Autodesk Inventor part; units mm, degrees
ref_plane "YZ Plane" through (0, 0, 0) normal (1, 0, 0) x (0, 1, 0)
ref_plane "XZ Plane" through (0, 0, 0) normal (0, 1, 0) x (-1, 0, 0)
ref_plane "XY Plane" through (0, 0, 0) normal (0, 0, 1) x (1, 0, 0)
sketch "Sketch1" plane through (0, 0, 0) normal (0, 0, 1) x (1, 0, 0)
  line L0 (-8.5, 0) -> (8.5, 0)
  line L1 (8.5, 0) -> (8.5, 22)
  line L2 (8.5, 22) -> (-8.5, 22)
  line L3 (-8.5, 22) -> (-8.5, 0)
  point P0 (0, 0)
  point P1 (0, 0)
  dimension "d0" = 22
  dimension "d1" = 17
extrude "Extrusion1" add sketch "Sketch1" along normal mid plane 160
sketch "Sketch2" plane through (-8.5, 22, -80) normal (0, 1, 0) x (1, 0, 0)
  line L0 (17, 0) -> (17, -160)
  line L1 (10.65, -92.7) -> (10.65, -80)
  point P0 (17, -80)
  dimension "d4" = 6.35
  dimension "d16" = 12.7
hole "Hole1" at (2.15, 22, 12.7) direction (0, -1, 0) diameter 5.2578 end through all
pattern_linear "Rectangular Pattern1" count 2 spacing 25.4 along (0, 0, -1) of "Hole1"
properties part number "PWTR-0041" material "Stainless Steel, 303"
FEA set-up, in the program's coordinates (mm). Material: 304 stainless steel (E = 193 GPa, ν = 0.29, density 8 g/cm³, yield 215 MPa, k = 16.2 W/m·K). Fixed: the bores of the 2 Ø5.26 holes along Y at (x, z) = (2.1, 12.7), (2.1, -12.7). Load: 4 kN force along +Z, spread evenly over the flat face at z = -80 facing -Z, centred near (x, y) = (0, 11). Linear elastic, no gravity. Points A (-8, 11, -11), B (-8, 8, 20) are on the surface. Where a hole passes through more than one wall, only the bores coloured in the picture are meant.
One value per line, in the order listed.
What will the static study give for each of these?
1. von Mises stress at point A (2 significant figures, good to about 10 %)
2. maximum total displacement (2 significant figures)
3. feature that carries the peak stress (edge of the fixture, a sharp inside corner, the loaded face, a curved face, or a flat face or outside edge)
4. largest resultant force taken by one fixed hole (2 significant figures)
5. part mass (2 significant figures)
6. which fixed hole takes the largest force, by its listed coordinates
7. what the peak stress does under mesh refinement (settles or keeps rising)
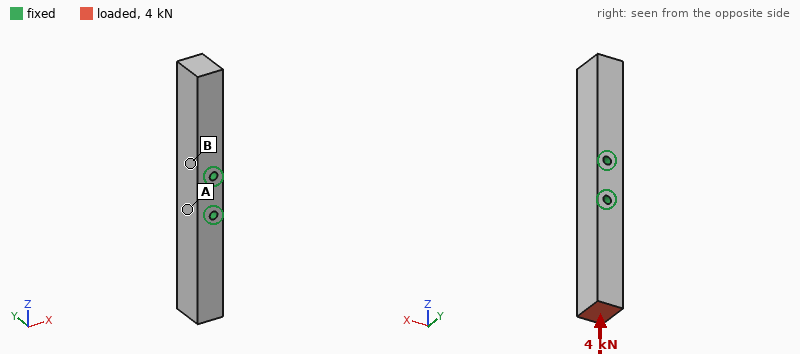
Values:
7.7 MPa
4.9 µm
edge of the fixture
3.6 kN
470 g
(2.1, -12.7)
keeps rising
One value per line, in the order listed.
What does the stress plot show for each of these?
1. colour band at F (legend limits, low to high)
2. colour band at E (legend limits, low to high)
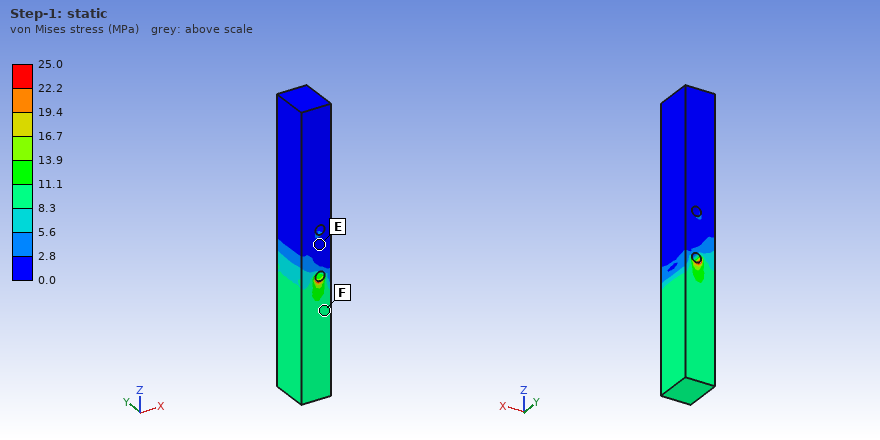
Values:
8.3 to 11.1 MPa
0.0 to 2.8 MPa
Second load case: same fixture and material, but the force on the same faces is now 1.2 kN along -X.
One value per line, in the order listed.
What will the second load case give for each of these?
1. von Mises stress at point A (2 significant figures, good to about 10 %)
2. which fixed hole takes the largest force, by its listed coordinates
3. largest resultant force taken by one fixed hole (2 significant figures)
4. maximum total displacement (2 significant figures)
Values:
48 MPa
(2.1, -12.7)
3.3 kN
89 µm
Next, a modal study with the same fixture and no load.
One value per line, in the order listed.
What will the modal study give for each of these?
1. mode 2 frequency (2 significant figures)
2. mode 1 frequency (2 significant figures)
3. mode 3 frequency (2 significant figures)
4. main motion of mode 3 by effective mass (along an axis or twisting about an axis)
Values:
2600 Hz
2500 Hz
3500 Hz
twisting about X
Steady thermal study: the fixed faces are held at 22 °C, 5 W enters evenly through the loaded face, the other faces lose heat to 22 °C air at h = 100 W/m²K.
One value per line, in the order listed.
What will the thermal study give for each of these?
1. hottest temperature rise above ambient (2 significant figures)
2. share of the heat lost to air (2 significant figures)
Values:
23 K
82 %
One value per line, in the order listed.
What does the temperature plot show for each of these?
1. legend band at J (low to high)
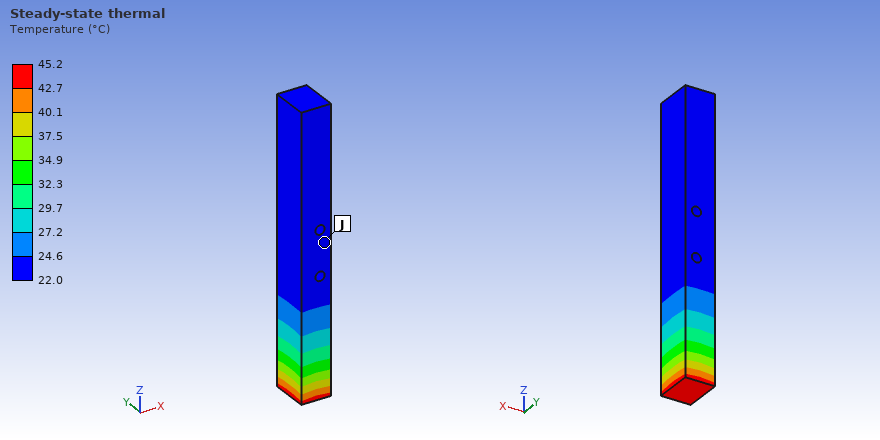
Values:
22.0 to 24.6 °C
